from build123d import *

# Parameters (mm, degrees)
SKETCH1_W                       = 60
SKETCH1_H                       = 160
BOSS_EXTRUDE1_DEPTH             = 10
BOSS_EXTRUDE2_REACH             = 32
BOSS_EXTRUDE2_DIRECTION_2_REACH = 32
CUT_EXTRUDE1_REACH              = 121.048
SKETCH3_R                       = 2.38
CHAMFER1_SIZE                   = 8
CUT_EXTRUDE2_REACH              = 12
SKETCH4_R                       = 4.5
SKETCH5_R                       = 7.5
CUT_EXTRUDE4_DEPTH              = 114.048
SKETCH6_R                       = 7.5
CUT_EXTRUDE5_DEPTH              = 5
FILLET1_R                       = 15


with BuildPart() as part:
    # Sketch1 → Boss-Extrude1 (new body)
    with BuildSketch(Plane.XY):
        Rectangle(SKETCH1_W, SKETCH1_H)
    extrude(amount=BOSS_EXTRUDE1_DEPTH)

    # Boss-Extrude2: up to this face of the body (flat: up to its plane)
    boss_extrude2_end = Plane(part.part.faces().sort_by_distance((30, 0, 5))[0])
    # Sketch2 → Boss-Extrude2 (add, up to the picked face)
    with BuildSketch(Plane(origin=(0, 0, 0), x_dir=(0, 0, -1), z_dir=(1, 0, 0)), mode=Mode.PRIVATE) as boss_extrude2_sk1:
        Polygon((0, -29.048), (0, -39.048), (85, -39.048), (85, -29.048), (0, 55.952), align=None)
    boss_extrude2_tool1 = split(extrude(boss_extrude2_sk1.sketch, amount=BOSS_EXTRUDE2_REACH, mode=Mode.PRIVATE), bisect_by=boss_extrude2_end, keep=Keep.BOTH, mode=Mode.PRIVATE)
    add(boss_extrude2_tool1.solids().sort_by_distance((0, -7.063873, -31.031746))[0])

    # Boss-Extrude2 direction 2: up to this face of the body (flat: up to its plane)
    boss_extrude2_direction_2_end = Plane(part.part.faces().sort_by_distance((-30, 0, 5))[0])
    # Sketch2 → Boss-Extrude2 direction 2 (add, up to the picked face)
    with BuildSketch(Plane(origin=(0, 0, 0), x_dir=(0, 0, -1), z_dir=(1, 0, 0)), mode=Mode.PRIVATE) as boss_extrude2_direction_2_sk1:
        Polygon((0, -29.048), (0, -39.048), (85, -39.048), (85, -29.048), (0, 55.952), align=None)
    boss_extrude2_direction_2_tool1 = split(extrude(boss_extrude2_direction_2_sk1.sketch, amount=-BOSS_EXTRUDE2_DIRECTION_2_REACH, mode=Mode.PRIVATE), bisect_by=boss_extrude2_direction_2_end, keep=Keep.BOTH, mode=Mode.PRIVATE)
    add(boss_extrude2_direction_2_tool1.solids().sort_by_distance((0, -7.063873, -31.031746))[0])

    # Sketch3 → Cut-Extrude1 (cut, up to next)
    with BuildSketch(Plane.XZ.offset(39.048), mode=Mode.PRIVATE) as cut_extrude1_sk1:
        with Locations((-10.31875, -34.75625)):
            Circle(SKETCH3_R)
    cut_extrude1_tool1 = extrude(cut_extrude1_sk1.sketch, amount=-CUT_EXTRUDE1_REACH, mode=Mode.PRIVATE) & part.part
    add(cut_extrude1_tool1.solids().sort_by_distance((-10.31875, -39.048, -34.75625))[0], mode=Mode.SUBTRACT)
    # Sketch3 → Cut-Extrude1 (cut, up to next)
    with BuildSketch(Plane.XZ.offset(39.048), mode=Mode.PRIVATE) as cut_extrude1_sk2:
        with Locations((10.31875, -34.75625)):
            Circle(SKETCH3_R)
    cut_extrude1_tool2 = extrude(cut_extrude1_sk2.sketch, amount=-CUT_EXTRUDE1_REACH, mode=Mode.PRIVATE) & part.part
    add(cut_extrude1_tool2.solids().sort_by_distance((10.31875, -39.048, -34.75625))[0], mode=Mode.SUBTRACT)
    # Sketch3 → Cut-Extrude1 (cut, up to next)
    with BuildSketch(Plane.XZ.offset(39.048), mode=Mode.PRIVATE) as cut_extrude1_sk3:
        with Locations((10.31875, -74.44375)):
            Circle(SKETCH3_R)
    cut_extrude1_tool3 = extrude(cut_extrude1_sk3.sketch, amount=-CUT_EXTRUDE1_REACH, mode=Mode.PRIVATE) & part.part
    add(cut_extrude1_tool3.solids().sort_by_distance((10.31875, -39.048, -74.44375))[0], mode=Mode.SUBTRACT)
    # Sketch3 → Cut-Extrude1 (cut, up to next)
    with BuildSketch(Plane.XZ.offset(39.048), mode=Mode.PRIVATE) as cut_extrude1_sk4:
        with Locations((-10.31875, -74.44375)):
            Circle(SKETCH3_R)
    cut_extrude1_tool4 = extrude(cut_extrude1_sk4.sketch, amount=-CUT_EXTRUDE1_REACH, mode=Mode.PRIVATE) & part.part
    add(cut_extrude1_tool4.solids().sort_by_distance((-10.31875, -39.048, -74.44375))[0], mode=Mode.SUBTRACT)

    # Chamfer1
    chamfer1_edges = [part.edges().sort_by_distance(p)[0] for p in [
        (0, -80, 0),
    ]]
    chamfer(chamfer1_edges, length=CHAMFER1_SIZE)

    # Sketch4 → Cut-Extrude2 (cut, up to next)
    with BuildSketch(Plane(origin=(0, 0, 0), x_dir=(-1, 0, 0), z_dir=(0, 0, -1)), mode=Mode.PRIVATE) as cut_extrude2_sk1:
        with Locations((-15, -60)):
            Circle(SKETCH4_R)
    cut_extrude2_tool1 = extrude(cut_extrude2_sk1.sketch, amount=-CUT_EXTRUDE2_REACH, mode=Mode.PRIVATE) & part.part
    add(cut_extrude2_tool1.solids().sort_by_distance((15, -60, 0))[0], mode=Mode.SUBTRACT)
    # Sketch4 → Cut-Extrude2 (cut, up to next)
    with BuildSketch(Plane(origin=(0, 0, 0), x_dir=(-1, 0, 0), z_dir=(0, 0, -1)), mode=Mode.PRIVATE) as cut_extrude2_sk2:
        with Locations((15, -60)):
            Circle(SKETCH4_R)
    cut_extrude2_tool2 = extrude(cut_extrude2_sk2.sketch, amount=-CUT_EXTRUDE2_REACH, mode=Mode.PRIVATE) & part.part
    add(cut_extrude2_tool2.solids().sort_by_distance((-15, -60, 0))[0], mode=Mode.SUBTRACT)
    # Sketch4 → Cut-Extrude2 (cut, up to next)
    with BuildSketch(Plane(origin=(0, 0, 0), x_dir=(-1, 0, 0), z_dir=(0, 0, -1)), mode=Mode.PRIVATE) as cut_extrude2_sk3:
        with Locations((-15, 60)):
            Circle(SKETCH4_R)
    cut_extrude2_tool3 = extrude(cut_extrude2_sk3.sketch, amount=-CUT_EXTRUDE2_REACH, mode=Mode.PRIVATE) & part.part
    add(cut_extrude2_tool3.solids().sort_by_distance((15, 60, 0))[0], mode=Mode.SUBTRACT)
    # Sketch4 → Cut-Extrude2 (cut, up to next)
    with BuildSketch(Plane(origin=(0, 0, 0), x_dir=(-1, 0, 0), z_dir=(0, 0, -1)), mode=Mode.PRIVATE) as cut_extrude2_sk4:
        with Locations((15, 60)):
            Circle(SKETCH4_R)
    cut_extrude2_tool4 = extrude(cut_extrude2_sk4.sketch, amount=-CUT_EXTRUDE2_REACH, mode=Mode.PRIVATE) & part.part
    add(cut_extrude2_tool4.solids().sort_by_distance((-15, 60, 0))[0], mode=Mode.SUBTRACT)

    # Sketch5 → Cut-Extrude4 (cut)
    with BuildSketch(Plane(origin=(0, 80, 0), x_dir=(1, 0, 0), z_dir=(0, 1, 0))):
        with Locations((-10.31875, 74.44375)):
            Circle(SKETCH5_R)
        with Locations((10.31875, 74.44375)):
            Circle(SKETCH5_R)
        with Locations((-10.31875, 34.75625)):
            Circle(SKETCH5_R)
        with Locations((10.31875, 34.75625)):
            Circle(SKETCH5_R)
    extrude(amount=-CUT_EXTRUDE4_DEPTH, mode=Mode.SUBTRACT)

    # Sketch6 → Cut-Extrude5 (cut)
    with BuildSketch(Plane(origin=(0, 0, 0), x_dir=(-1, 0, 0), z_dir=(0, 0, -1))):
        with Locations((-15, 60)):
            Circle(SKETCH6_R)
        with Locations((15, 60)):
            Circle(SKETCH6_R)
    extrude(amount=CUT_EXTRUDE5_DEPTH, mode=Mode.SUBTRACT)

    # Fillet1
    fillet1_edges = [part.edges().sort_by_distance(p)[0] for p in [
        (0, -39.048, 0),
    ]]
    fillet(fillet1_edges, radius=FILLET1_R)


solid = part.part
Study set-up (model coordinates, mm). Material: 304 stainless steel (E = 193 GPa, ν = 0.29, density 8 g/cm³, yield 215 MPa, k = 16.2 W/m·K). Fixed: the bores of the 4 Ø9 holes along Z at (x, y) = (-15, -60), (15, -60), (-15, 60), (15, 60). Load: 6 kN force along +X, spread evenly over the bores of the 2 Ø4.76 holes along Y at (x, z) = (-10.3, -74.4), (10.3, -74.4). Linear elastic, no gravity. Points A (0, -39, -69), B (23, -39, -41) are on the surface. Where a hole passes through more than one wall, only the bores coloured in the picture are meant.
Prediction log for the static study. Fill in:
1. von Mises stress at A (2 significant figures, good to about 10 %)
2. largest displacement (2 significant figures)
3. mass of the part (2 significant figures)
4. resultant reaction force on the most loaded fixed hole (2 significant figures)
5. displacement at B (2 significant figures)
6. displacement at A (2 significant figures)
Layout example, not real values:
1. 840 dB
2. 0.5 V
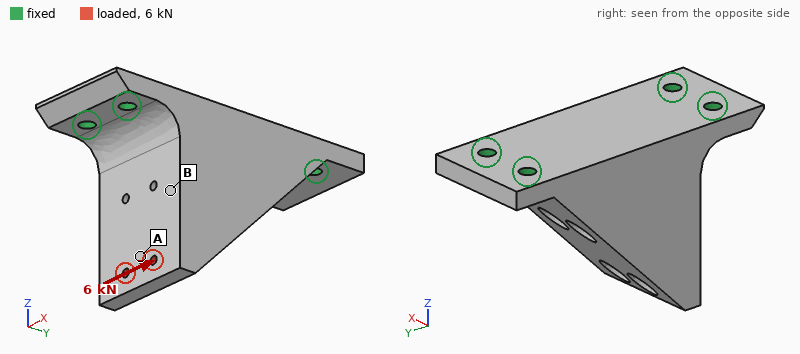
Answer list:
1. 31 MPa
2. 76 µm
3. 2.7 kg
4. 9.5 kN
5. 40 µm
6. 60 µm
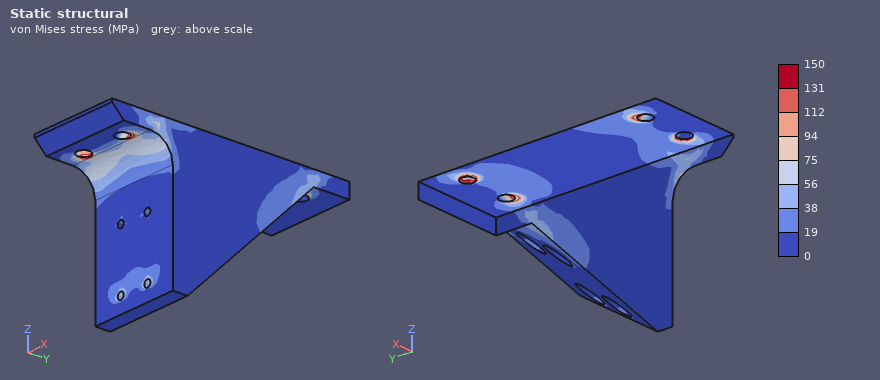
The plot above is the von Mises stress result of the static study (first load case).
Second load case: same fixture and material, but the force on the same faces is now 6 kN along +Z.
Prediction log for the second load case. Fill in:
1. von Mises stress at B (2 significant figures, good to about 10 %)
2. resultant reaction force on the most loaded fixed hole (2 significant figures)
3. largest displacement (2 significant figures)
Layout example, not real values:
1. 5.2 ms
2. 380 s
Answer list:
1. 9.8 MPa
2. 2.8 kN
3. 14 µm
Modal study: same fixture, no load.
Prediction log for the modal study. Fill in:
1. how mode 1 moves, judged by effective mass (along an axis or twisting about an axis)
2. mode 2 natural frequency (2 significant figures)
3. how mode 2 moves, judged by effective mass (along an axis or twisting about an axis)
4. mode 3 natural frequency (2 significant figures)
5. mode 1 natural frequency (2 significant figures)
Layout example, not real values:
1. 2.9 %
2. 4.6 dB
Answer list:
1. along X
2. 4100 Hz
3. along Z
4. 5500 Hz
5. 2000 Hz
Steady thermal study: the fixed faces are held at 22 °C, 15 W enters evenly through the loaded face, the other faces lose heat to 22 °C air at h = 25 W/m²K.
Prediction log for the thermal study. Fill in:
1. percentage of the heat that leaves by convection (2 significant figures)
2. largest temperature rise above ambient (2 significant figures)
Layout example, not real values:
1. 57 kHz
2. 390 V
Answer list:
1. 69 %
2. 55 K
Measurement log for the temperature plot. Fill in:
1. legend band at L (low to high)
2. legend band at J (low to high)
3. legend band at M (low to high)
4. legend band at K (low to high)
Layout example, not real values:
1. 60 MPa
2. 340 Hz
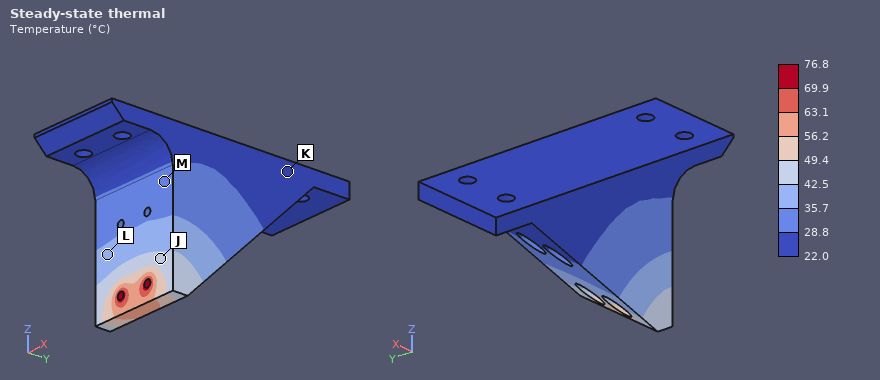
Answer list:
1. 35.7 to 42.5 °C
2. 42.5 to 49.4 °C
3. 28.8 to 35.7 °C
4. 22.0 to 28.8 °C
